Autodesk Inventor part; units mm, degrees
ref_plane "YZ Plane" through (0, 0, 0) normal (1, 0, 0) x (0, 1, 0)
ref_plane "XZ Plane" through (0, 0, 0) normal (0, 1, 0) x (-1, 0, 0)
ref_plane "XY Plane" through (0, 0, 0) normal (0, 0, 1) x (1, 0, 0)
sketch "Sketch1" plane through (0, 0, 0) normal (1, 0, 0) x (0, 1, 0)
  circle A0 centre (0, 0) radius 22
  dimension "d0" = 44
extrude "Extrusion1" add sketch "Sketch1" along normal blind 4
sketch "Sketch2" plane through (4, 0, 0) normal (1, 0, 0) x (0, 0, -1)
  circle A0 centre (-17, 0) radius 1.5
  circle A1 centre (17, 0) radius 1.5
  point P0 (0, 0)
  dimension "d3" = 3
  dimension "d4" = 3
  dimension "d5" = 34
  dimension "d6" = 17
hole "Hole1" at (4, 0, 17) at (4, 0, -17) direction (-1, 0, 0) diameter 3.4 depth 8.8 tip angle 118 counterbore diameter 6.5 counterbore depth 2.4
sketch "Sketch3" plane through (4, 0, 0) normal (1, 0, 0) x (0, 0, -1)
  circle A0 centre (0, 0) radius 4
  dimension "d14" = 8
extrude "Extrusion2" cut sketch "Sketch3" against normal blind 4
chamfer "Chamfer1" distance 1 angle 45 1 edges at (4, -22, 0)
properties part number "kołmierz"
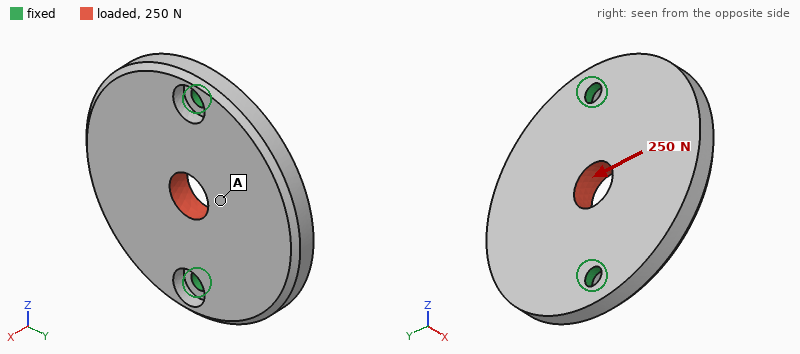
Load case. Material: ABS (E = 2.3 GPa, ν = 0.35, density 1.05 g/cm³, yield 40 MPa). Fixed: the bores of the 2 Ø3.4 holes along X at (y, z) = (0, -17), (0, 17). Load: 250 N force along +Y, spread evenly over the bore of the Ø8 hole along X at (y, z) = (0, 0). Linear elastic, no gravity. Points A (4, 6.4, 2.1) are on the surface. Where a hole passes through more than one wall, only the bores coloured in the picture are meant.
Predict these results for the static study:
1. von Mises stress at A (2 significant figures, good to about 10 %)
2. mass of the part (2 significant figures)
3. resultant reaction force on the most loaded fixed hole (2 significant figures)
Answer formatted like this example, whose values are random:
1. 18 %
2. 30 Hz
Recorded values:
1. 2.1 MPa
2. 5.9 g
3. 130 N
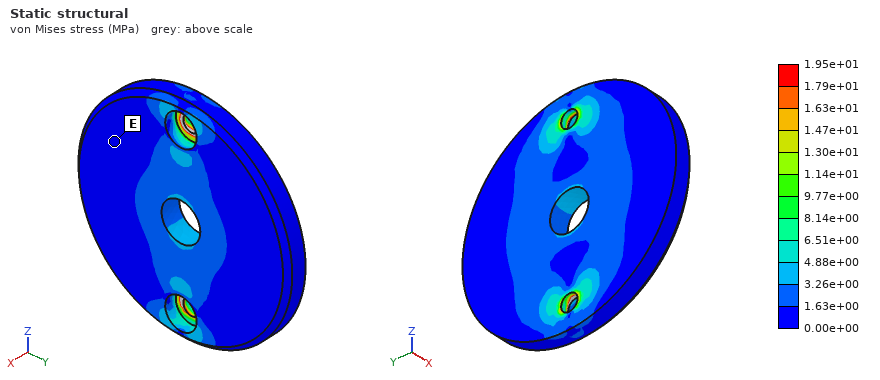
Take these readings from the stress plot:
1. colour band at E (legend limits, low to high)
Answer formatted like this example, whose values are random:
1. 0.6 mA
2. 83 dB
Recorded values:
1. 0.00e+00 to 1.63e+00 MPa
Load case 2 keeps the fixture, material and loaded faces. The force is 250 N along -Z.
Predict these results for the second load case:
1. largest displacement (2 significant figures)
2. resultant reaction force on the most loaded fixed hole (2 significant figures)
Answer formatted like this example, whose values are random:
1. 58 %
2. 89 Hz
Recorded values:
1. 28 µm
2. 130 N
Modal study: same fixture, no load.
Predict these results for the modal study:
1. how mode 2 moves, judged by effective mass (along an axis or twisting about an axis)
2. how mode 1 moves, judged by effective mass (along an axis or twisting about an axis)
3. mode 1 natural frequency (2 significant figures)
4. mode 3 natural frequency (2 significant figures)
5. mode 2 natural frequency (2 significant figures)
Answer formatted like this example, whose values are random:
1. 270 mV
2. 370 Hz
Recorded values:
1. along X
2. twisting about Z
3. 980 Hz
4. 3500 Hz
5. 1800 Hz
